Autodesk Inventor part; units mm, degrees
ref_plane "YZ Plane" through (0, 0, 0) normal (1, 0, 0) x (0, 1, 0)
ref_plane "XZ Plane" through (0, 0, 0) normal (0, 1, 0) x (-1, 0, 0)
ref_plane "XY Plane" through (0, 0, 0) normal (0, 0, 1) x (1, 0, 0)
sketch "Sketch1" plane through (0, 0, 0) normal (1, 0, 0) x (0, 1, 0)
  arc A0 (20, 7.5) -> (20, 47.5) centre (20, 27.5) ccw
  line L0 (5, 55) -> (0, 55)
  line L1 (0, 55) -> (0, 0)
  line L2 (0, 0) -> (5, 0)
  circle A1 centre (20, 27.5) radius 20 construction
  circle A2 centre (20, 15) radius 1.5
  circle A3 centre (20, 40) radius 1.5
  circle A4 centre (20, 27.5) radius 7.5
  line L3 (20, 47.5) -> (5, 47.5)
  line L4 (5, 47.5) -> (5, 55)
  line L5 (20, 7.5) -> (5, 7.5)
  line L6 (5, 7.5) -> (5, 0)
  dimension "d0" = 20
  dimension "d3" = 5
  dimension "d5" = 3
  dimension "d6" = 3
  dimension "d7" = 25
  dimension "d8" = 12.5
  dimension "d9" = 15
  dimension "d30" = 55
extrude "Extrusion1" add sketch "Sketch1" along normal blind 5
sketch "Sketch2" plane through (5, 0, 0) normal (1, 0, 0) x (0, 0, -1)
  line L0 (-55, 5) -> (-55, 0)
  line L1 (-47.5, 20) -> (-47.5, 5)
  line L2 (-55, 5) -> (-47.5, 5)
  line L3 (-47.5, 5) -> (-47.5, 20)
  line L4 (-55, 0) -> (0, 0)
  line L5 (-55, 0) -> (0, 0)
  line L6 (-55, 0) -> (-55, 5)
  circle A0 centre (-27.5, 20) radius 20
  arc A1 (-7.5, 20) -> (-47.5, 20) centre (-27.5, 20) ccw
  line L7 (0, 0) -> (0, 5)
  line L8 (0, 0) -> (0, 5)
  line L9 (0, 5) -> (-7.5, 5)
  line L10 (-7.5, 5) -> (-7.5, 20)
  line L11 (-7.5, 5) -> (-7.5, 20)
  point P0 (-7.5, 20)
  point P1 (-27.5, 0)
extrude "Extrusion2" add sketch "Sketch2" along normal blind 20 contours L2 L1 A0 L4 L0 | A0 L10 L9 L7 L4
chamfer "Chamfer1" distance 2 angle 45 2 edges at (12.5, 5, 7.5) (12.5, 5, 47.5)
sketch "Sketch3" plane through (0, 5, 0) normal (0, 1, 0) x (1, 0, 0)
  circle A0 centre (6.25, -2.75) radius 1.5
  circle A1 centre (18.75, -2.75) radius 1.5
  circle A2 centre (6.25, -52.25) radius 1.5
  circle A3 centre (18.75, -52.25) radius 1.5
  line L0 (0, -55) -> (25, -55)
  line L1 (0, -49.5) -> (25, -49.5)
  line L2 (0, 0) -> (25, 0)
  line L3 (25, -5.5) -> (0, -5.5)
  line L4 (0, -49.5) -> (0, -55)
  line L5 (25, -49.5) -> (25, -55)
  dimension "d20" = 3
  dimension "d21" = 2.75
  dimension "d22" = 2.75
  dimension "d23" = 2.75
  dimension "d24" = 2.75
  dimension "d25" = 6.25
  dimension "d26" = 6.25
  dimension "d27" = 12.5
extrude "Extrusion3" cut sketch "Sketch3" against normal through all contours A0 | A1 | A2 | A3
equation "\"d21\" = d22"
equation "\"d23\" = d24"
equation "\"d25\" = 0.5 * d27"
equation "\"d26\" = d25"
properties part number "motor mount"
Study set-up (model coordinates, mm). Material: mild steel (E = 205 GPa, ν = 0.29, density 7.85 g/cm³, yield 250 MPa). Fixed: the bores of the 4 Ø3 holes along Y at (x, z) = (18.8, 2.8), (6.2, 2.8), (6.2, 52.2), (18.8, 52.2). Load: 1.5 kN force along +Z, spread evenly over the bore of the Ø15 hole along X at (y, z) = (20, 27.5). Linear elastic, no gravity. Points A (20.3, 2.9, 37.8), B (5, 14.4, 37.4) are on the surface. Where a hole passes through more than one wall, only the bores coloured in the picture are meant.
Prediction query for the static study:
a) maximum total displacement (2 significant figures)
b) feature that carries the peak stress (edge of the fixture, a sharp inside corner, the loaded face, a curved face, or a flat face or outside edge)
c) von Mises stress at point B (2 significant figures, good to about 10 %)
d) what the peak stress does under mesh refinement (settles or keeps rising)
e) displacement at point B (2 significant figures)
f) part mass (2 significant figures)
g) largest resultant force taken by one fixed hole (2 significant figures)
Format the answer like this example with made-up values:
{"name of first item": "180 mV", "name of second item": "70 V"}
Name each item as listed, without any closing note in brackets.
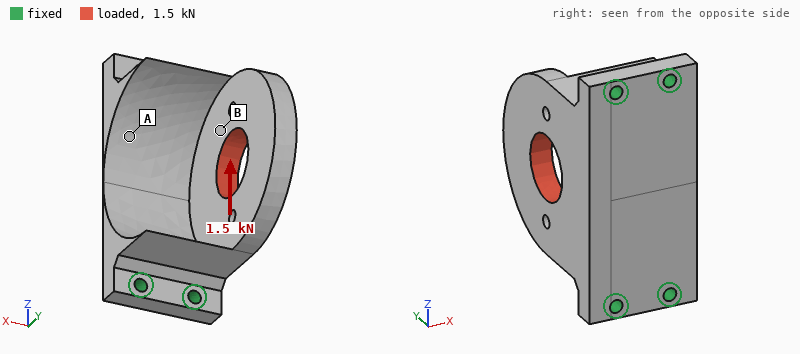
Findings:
{"maximum total displacement": "8.0 µm", "feature that carries the peak stress": "edge of the fixture", "von Mises stress at point B": "15 MPa", "what the peak stress does under mesh refinement": "keeps rising", "displacement at point B": "3.2 µm", "part mass": "90 g", "largest resultant force taken by one fixed hole": "980 N"}
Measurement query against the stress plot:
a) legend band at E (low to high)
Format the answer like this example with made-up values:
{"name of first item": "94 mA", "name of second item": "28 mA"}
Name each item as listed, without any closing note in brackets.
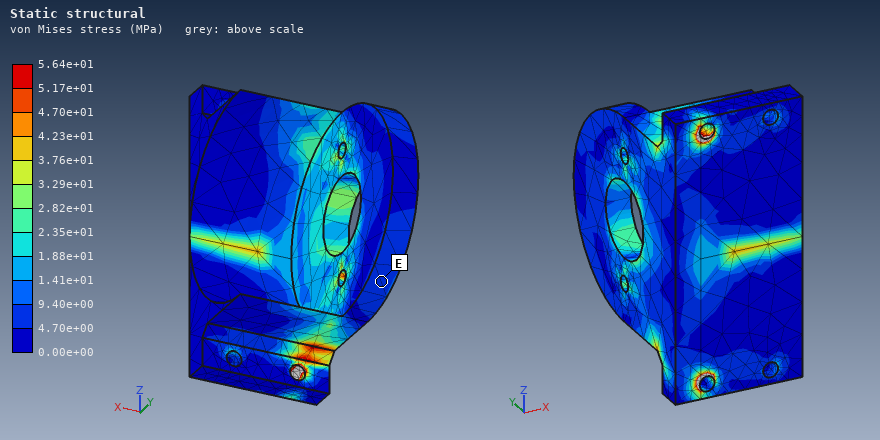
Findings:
{"legend band at E": "4.70e+00 to 9.40e+00 MPa"}
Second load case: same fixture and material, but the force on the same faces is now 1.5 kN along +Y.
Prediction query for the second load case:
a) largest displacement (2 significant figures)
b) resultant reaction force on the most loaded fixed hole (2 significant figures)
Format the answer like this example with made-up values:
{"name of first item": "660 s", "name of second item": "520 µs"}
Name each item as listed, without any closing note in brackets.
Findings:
{"largest displacement": "12 µm", "resultant reaction force on the most loaded fixed hole": "940 N"}
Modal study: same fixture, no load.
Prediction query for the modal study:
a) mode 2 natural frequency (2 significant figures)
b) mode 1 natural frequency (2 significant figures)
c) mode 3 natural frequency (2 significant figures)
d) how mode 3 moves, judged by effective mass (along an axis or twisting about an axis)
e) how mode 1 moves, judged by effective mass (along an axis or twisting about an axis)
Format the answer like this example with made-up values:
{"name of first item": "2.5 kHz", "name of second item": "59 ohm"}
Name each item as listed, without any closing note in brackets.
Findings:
{"mode 2 natural frequency": "9900 Hz", "mode 1 natural frequency": "3600 Hz", "mode 3 natural frequency": "13 kHz", "how mode 3 moves, judged by effective mass": "along Y", "how mode 1 moves, judged by effective mass": "along X"}
